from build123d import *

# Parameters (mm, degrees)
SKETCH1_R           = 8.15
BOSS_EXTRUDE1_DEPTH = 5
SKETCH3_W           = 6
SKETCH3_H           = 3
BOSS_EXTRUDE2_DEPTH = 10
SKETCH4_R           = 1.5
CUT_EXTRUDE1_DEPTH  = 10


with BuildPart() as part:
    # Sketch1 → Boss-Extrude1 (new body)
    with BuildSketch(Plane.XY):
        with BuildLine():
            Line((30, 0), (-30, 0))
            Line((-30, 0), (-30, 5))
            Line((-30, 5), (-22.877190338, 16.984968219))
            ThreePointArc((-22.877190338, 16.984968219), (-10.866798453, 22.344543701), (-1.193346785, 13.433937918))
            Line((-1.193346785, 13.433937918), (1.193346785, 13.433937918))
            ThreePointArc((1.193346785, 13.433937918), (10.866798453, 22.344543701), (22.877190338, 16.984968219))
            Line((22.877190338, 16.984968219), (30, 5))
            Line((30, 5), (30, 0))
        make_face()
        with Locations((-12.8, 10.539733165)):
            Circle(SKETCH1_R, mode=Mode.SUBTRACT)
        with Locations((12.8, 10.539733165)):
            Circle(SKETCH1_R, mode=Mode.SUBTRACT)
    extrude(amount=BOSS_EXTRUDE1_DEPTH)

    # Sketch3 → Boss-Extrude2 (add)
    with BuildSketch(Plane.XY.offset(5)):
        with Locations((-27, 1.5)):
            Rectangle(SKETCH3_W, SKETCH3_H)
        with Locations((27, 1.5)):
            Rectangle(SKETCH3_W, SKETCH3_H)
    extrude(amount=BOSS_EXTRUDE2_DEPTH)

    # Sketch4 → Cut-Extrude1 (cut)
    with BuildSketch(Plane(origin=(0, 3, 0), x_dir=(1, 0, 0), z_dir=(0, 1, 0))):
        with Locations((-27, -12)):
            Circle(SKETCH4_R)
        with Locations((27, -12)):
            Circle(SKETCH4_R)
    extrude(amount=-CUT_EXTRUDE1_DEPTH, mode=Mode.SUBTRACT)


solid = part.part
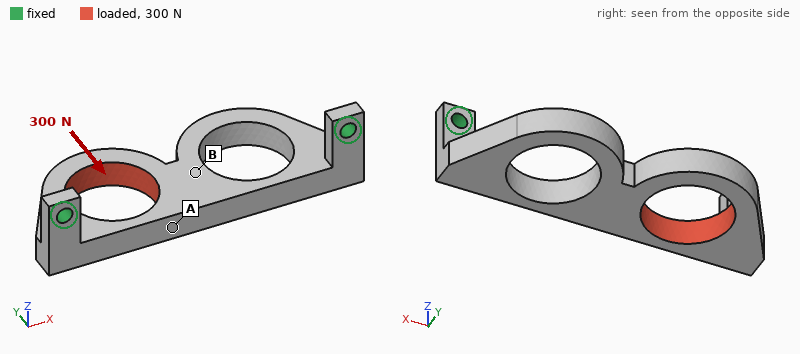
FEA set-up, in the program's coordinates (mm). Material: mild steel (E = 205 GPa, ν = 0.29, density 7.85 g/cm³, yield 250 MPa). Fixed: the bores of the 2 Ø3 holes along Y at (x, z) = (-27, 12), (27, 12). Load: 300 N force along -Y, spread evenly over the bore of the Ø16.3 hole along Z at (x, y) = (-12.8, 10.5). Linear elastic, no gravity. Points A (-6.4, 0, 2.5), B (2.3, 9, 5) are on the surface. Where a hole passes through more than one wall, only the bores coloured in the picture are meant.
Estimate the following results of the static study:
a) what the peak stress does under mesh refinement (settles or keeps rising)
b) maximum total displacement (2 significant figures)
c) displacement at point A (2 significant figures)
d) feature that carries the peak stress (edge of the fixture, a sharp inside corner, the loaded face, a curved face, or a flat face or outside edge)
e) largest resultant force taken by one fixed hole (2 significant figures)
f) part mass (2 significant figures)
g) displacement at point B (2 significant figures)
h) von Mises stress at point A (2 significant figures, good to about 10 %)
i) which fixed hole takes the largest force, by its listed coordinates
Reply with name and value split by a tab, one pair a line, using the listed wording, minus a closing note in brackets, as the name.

what the peak stress does under mesh refinement	keeps rising
maximum total displacement	51 µm
displacement at point A	23 µm
feature that carries the peak stress	edge of the fixture
largest resultant force taken by one fixed hole	220 N
part mass	28 g
displacement at point B	23 µm
von Mises stress at point A	28 MPa
which fixed hole takes the largest force, by its listed coordinates	(-27, 12)
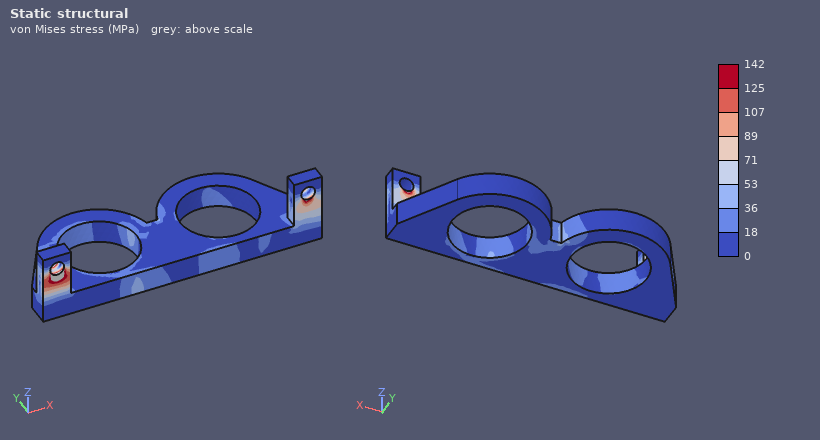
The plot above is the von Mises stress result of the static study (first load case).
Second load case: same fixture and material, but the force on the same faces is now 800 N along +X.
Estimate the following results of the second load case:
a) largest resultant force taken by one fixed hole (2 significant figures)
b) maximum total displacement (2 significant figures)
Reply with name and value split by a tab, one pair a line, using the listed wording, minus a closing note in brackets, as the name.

largest resultant force taken by one fixed hole	440 N
maximum total displacement	24 µm
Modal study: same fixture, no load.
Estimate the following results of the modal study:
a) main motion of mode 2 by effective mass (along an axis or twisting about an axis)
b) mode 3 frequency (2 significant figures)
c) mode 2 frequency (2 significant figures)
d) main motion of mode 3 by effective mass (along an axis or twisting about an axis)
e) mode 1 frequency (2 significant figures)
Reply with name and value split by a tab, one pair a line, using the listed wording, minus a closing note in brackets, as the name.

main motion of mode 2 by effective mass	along Y
mode 3 frequency	5900 Hz
mode 2 frequency	5500 Hz
main motion of mode 3 by effective mass	along X
mode 1 frequency	2200 Hz
